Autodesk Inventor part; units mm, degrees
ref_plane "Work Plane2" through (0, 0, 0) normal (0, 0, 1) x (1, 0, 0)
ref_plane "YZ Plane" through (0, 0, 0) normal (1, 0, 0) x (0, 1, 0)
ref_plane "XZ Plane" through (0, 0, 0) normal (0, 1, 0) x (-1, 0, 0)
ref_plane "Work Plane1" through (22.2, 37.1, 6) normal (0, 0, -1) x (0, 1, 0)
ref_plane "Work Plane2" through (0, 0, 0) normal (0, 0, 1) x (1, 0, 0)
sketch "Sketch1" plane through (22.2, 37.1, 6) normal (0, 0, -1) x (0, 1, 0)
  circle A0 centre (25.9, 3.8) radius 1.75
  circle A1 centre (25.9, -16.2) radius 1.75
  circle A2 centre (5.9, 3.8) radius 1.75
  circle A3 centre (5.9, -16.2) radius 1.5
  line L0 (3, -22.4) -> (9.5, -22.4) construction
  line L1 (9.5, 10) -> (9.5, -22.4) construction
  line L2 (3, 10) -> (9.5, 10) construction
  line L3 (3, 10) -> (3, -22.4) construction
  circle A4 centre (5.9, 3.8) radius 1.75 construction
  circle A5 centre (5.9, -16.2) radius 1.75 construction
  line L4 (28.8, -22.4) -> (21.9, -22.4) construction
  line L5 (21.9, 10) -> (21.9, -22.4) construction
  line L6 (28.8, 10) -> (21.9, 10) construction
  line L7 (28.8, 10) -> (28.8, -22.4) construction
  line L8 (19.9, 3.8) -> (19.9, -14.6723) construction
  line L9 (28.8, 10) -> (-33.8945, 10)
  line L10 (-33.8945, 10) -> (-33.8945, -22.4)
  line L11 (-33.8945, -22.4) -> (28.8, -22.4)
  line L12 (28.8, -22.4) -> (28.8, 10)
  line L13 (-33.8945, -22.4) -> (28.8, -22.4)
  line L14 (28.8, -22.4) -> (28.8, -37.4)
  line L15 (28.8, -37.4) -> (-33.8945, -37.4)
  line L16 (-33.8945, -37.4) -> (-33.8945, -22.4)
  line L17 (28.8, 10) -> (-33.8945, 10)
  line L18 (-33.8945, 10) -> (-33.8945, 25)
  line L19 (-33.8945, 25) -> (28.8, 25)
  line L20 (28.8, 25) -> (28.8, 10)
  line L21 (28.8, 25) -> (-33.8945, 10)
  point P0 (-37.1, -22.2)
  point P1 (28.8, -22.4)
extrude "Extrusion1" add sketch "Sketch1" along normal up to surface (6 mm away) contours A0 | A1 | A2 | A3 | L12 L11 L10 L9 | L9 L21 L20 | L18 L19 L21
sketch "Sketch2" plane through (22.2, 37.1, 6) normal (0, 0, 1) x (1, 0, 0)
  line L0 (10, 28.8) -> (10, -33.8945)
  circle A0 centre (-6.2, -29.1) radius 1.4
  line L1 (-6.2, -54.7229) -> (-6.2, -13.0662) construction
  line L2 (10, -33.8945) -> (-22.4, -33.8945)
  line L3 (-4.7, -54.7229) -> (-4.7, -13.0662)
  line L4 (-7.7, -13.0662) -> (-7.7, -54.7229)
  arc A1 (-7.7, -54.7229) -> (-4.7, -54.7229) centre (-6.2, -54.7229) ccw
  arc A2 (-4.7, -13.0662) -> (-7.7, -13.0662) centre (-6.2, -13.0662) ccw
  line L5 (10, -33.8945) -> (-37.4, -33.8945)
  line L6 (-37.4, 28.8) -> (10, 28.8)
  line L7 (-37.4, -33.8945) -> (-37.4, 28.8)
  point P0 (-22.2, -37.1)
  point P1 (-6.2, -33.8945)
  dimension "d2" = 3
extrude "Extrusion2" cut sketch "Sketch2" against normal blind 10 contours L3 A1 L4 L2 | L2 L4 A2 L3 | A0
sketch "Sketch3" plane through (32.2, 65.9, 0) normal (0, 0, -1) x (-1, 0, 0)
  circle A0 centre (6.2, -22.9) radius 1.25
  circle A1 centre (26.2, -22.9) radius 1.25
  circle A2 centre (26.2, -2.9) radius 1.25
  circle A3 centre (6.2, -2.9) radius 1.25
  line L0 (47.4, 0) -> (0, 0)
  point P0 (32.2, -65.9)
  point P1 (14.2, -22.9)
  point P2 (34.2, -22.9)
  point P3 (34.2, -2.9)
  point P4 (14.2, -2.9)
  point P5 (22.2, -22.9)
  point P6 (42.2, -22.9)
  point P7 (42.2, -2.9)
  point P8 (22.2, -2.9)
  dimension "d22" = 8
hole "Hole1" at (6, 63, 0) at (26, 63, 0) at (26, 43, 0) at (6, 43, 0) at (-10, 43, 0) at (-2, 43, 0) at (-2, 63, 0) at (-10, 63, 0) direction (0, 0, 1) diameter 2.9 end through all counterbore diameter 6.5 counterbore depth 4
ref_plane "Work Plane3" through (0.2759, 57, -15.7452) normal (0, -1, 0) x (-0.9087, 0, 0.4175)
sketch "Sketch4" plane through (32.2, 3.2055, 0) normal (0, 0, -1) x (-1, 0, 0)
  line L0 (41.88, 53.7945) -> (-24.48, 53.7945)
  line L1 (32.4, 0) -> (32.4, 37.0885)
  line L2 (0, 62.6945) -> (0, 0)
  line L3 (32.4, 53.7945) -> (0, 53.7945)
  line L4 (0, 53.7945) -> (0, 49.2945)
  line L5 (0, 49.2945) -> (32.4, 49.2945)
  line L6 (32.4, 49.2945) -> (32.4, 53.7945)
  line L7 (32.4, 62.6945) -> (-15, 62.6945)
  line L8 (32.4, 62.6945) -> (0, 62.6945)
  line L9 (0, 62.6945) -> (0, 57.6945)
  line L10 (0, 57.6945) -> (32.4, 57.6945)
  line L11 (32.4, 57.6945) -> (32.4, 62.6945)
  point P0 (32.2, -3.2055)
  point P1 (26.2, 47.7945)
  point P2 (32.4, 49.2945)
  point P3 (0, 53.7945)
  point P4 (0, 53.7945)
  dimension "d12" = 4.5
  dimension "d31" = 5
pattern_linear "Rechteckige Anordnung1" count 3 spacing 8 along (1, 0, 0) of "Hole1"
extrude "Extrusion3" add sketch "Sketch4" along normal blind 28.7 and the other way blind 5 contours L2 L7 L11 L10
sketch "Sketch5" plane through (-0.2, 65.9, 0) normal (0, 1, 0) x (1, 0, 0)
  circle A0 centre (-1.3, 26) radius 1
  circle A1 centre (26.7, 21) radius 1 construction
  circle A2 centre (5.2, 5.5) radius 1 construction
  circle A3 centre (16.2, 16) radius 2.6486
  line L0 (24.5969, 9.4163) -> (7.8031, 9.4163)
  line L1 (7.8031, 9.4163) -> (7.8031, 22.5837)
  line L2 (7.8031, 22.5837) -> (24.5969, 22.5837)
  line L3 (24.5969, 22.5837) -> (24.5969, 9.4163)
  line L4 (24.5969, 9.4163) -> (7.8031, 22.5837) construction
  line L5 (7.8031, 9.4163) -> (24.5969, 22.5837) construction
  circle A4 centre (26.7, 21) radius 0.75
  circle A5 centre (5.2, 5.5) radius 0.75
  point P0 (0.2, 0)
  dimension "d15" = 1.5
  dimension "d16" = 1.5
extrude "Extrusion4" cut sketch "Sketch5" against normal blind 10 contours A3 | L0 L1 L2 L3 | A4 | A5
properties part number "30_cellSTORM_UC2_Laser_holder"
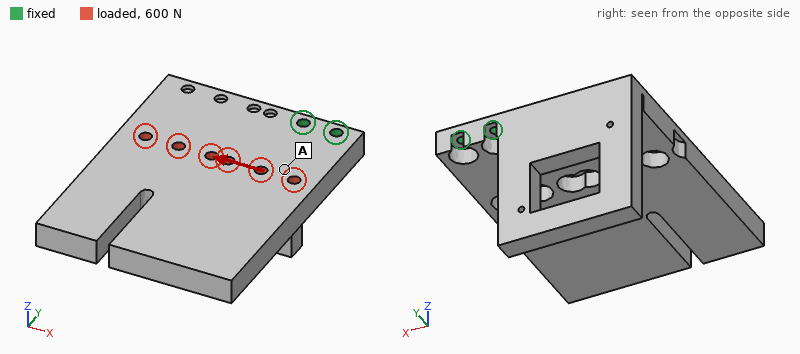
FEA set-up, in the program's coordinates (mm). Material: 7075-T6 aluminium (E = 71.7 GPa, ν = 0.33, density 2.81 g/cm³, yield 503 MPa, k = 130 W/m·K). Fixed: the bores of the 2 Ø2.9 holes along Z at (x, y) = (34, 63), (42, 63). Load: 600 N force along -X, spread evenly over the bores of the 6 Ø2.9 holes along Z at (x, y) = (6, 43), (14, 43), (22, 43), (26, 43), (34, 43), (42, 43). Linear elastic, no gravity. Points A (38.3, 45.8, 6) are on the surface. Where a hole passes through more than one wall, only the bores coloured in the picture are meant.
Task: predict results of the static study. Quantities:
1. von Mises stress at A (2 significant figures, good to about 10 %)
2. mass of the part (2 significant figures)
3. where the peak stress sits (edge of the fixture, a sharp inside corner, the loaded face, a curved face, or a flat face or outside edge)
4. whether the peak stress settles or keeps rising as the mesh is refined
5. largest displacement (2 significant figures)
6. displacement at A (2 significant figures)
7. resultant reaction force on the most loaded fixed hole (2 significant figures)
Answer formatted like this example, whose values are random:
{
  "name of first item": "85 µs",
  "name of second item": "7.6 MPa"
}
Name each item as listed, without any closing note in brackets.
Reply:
{
  "von Mises stress at A": "17 MPa",
  "mass of the part": "55 g",
  "where the peak stress sits": "edge of the fixture",
  "whether the peak stress settles or keeps rising as the mesh is refined": "keeps rising",
  "largest displacement": "0.13 mm",
  "displacement at A": "0.029 mm",
  "resultant reaction force on the most loaded fixed hole": "1.1 kN"
}
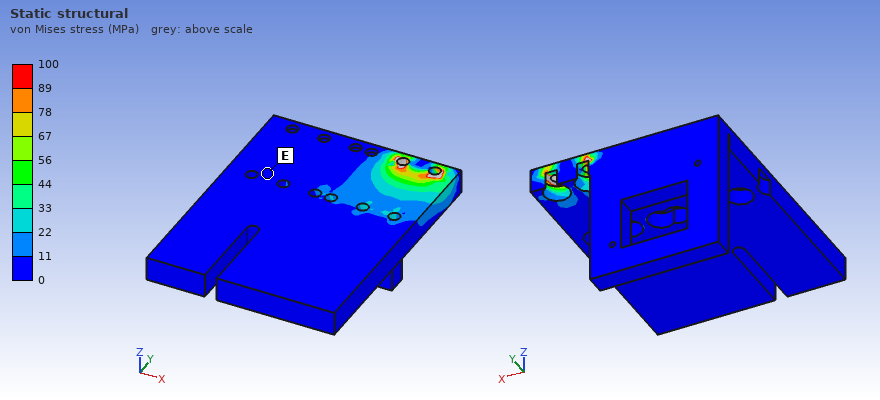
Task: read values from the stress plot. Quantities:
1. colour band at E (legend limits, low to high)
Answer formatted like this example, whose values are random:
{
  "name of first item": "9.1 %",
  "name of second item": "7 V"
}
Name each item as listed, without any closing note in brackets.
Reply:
{
  "colour band at E": "0 to 11 MPa"
}
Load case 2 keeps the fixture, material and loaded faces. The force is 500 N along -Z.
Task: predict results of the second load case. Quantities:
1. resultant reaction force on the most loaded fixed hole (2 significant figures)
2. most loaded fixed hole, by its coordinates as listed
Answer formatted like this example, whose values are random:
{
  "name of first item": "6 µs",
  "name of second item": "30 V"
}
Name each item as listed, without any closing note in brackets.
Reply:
{
  "resultant reaction force on the most loaded fixed hole": "900 N",
  "most loaded fixed hole, by its coordinates as listed": "(34, 63)"
}
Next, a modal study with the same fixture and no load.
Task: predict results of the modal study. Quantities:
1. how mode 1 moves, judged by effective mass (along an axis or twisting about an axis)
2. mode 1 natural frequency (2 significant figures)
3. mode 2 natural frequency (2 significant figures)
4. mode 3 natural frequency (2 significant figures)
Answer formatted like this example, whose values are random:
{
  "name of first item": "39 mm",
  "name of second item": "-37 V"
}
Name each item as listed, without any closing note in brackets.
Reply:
{
  "how mode 1 moves, judged by effective mass": "along Z",
  "mode 1 natural frequency": "570 Hz",
  "mode 2 natural frequency": "1300 Hz",
  "mode 3 natural frequency": "1600 Hz"
}
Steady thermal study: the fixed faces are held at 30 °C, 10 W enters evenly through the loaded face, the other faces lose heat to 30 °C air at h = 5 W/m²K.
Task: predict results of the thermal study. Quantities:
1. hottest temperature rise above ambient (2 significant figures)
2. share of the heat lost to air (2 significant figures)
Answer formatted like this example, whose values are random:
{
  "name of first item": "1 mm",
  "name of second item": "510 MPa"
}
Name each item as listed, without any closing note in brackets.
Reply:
{
  "hottest temperature rise above ambient": "16 K",
  "share of the heat lost to air": "5.6 %"
}
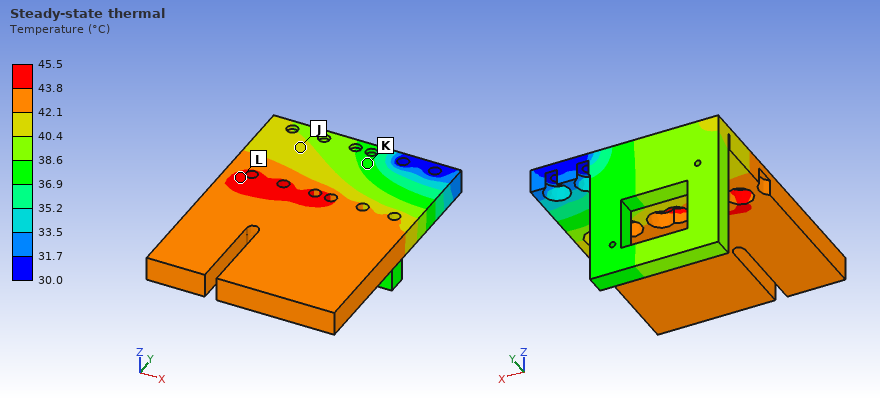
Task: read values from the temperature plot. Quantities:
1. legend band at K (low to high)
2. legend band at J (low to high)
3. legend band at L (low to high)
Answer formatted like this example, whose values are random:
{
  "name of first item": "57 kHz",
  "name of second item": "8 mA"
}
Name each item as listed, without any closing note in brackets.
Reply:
{
  "legend band at K": "36.9 to 38.6 °C",
  "legend band at J": "40.4 to 42.1 °C",
  "legend band at L": "43.8 to 45.5 °C"
}
